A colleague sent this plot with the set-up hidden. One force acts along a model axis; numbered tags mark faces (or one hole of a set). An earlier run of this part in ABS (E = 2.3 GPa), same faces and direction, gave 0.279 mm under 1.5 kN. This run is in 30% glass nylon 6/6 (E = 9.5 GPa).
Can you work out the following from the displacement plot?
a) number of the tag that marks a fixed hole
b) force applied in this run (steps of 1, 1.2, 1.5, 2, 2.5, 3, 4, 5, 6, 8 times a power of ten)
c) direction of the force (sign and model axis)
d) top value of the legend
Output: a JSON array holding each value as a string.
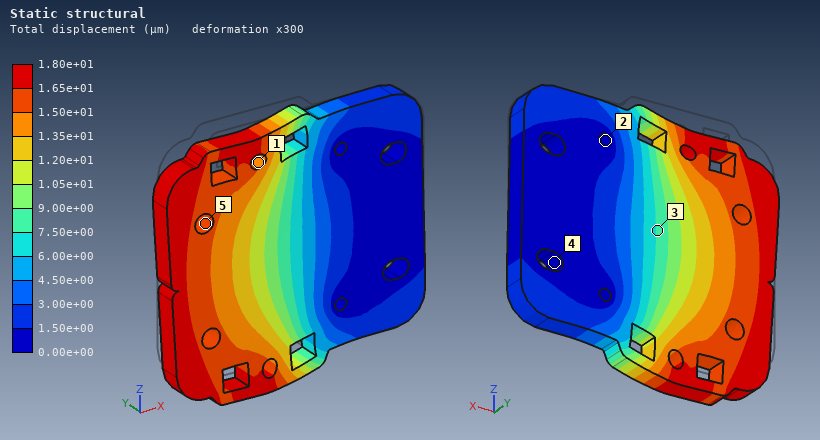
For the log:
["2", "400 N", "-Z", "1.80e+01 µm"]
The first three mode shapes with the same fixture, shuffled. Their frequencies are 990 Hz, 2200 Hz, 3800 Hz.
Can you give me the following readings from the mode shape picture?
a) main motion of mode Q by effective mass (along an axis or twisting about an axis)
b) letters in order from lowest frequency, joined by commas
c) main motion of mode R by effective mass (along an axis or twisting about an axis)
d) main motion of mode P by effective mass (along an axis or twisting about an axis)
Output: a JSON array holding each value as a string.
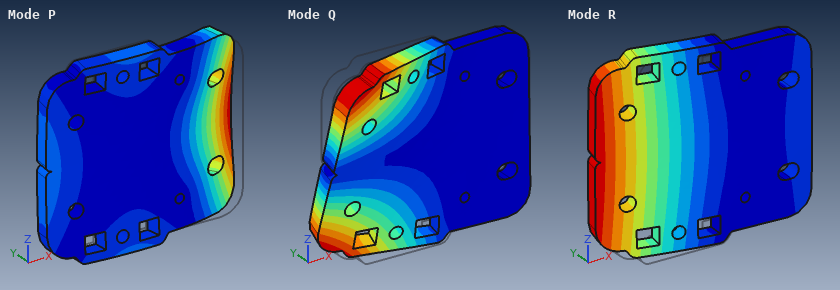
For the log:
["twisting about X", "R, Q, P", "along Y", "along Y"]
